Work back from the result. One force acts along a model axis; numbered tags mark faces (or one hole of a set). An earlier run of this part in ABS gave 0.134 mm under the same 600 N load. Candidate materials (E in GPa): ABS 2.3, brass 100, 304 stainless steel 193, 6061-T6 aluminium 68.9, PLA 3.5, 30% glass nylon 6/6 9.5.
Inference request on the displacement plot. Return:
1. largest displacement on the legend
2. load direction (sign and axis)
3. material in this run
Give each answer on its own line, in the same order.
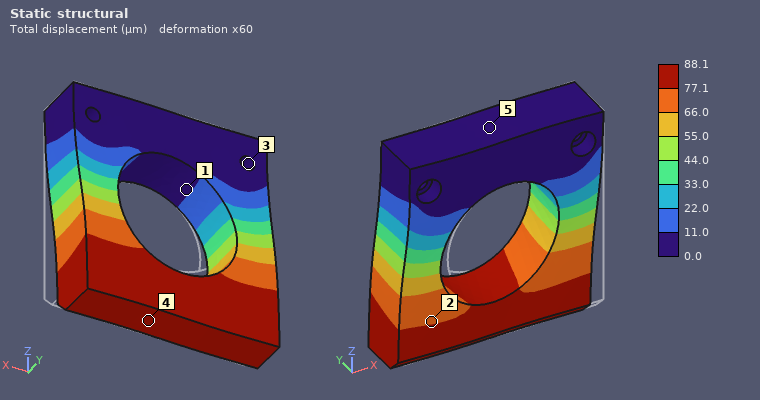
88.1 µm
-X
PLA
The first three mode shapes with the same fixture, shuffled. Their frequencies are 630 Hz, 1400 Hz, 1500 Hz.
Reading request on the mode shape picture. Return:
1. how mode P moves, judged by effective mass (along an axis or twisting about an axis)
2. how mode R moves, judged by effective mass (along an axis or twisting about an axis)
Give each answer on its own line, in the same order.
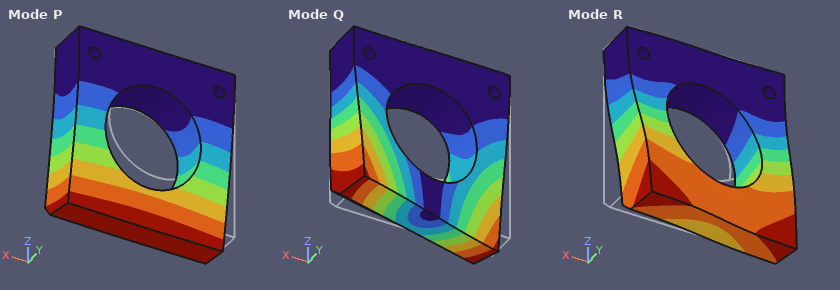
along Y
along X
